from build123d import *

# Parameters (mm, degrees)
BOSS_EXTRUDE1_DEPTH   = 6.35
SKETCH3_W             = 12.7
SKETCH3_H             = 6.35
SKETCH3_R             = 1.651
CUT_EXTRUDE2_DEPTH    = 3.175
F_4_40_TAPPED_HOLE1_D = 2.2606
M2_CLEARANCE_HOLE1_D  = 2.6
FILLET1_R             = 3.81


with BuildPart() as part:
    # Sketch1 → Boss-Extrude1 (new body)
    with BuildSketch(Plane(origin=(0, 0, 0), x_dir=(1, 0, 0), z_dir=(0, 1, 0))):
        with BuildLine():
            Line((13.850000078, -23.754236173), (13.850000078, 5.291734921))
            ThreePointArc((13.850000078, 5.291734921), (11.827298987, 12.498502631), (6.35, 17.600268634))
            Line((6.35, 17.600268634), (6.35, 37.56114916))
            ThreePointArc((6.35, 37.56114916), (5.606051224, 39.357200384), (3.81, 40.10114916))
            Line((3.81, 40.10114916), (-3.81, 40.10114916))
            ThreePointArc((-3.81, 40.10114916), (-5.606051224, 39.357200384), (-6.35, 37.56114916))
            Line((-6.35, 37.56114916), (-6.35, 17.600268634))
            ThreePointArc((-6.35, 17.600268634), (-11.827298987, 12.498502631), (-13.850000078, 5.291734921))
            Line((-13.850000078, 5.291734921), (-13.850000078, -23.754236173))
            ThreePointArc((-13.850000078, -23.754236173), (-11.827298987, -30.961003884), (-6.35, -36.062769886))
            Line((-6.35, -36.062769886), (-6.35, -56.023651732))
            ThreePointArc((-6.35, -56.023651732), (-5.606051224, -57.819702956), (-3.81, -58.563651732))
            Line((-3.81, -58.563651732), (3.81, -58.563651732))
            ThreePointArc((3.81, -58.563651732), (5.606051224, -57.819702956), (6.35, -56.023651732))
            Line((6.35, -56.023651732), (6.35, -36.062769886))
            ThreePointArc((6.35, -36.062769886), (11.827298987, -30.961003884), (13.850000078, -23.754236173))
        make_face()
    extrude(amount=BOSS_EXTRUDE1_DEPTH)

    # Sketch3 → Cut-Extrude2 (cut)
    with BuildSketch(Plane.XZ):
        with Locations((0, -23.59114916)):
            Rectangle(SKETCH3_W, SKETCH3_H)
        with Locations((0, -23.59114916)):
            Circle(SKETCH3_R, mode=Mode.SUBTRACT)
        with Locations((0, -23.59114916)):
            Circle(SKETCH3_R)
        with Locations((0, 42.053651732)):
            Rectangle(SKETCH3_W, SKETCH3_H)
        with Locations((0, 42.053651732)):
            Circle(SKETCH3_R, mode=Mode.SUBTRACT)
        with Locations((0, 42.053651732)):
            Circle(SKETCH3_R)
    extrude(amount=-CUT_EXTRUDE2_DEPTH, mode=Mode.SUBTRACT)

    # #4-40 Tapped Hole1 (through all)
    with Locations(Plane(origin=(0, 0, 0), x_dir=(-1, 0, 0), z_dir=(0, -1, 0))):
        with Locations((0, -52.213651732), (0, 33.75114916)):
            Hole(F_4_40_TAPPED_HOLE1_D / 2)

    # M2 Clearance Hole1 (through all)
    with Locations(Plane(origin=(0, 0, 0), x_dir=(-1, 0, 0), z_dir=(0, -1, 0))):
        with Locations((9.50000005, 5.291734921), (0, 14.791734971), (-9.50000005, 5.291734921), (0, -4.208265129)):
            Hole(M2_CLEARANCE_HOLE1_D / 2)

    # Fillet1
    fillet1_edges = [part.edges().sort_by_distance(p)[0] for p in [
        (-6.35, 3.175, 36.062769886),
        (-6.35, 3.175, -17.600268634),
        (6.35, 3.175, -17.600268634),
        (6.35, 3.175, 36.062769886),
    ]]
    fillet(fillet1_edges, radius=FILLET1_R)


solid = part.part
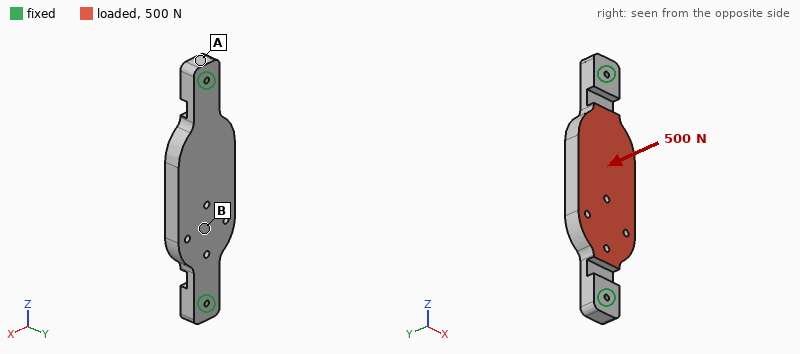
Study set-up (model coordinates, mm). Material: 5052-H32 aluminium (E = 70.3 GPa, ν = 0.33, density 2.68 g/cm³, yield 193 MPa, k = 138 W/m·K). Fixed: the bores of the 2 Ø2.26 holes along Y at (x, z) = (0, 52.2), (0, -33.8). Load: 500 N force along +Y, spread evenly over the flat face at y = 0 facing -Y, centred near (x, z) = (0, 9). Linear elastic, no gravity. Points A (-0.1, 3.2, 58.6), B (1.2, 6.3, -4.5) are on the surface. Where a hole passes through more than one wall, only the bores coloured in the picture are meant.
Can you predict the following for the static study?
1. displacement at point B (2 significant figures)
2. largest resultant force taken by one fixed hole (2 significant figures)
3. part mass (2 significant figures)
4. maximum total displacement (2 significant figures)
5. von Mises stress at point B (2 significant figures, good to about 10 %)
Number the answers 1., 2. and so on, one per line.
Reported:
1. 55 µm
2. 360 N
3. 31 g
4. 67 µm
5. 18 MPa
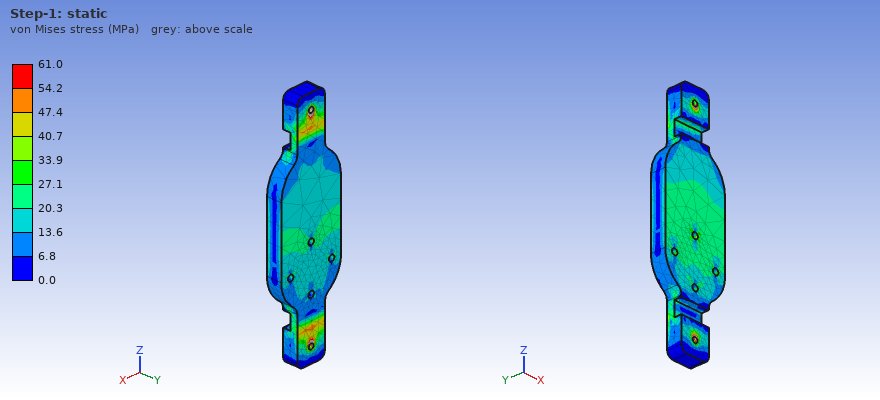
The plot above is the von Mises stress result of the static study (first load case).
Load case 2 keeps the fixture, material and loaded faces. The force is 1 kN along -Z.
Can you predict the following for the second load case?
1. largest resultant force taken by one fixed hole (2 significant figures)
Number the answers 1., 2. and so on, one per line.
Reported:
1. 510 N
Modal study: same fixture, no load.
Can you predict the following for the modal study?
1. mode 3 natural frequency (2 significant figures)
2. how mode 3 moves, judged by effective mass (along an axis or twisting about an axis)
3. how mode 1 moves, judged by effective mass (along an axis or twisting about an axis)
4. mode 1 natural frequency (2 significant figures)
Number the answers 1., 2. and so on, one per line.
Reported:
1. 6200 Hz
2. along X
3. along Y
4. 3000 Hz
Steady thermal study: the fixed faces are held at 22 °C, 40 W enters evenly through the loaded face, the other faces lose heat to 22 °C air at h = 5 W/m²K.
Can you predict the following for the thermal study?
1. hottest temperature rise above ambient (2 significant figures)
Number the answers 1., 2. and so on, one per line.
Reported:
1. 62 K
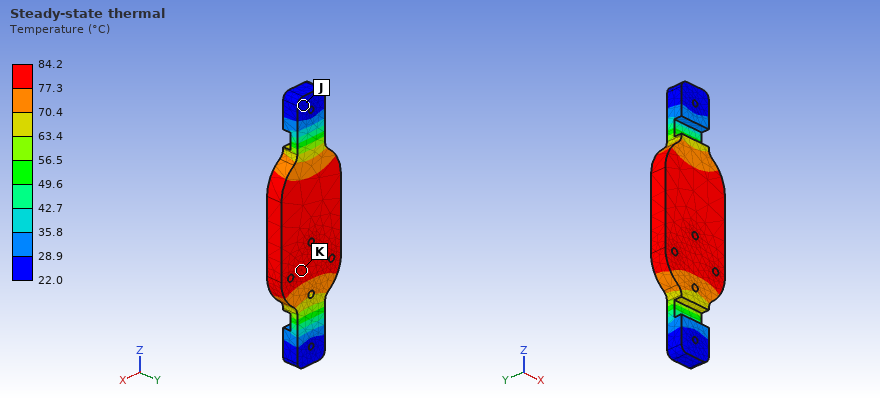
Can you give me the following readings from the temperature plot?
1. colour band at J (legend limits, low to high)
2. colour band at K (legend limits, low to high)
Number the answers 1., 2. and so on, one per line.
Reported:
1. 22.0 to 28.9 °C
2. 77.3 to 84.2 °C
